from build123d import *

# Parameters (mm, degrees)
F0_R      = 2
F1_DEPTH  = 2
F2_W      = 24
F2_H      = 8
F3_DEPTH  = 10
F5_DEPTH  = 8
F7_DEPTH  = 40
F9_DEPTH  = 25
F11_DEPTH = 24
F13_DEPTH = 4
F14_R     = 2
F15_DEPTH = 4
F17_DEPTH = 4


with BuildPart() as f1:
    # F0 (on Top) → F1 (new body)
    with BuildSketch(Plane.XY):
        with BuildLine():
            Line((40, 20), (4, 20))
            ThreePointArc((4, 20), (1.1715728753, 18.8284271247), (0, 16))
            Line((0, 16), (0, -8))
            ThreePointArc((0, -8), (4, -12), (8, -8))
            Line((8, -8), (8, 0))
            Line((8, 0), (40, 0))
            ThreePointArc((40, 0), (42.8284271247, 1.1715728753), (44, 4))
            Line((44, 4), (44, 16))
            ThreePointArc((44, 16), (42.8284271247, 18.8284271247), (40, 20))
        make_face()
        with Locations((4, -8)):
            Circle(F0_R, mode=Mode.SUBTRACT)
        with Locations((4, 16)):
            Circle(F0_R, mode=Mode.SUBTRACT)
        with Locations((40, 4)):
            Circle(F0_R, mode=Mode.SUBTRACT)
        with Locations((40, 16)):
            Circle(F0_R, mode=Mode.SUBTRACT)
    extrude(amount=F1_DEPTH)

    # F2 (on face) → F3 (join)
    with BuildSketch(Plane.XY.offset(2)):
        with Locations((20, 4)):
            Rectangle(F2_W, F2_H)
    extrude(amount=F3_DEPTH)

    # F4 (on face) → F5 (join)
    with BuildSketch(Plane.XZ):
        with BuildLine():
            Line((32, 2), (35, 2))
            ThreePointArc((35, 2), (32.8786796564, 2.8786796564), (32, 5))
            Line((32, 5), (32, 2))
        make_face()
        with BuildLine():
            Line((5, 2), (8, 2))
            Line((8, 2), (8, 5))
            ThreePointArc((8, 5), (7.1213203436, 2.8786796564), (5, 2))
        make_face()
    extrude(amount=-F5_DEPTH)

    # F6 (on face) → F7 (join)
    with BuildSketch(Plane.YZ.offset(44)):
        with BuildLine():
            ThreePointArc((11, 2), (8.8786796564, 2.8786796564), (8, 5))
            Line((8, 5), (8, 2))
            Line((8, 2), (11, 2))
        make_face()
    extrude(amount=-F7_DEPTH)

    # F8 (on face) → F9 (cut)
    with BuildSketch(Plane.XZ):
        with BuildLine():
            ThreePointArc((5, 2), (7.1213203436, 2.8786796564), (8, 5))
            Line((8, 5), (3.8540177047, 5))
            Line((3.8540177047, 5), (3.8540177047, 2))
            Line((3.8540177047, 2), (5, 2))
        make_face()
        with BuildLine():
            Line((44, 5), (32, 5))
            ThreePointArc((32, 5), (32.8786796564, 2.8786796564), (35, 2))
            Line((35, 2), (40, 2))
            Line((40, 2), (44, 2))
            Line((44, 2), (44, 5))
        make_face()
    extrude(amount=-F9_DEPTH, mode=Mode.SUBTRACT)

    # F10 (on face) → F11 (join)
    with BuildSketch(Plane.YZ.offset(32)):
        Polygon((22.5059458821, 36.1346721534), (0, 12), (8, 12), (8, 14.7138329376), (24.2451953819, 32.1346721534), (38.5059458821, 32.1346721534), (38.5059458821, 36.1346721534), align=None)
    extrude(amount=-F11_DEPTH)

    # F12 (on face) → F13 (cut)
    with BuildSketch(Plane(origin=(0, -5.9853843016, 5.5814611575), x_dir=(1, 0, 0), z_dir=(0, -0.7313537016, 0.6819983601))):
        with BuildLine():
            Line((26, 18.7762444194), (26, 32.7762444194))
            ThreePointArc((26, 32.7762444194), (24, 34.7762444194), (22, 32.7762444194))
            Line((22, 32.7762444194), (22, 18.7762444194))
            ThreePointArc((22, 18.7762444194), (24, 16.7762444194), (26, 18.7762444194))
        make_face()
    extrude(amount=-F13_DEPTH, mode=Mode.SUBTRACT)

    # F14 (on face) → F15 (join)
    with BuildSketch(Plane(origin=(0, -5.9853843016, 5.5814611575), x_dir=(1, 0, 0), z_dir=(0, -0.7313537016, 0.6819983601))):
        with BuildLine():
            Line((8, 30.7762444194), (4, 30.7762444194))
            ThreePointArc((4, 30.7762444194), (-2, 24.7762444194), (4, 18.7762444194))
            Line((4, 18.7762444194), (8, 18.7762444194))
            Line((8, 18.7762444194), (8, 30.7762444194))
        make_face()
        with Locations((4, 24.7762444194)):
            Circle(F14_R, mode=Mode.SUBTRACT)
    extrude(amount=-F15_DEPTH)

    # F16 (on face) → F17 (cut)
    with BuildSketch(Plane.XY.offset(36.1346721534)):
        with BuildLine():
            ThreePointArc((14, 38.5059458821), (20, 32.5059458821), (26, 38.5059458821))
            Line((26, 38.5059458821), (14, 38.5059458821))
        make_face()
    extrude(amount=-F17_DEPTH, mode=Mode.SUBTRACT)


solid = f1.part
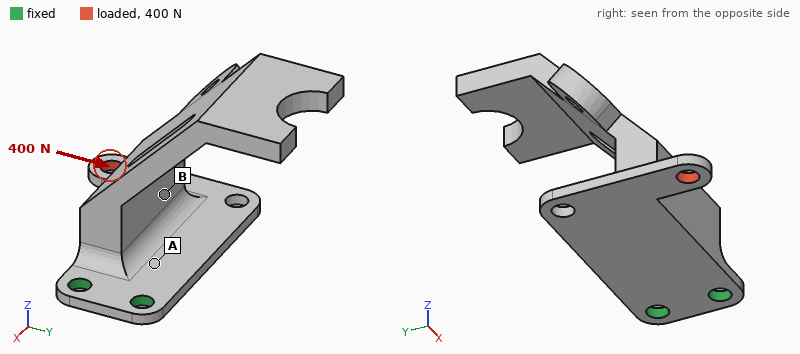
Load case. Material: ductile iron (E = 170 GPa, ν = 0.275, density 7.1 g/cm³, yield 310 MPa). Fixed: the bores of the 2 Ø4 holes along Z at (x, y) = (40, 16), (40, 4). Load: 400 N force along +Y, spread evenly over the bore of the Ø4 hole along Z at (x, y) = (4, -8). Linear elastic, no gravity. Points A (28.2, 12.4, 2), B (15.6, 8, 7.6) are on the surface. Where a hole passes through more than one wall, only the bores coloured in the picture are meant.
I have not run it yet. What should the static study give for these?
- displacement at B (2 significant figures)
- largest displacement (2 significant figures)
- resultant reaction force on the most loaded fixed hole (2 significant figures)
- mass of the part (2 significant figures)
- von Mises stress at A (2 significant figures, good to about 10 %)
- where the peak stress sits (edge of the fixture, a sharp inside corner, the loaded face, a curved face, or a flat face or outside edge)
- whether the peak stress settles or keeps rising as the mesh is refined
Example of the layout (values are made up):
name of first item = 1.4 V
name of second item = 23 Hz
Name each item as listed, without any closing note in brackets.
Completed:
displacement at B = 15 µm
largest displacement = 43 µm
resultant reaction force on the most loaded fixed hole = 1.0 kN
mass of the part = 58 g
von Mises stress at A = 36 MPa
where the peak stress sits = edge of the fixture
whether the peak stress settles or keeps rising as the mesh is refined = keeps rising
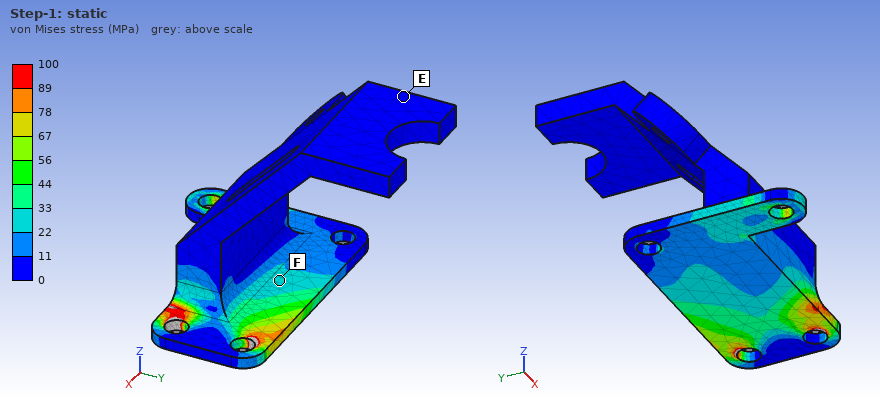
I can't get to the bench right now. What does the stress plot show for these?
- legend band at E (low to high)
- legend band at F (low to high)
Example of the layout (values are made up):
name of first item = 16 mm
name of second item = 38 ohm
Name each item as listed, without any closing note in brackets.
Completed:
legend band at E = 0 to 11 MPa
legend band at F = 22 to 33 MPa
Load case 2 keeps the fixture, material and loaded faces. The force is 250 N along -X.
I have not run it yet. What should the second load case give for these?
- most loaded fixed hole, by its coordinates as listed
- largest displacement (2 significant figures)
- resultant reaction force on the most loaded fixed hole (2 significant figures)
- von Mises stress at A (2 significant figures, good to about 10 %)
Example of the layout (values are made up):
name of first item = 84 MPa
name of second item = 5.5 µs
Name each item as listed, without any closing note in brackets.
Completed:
most loaded fixed hole, by its coordinates as listed = (40, 4)
largest displacement = 36 µm
resultant reaction force on the most loaded fixed hole = 450 N
von Mises stress at A = 7.2 MPa
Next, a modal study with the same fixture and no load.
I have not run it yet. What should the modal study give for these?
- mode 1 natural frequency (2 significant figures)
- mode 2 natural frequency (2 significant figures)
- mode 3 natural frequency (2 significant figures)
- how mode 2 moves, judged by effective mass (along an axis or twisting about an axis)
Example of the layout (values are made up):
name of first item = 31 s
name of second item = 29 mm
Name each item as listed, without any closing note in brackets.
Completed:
mode 1 natural frequency = 440 Hz
mode 2 natural frequency = 840 Hz
mode 3 natural frequency = 3500 Hz
how mode 2 moves, judged by effective mass = along Y
